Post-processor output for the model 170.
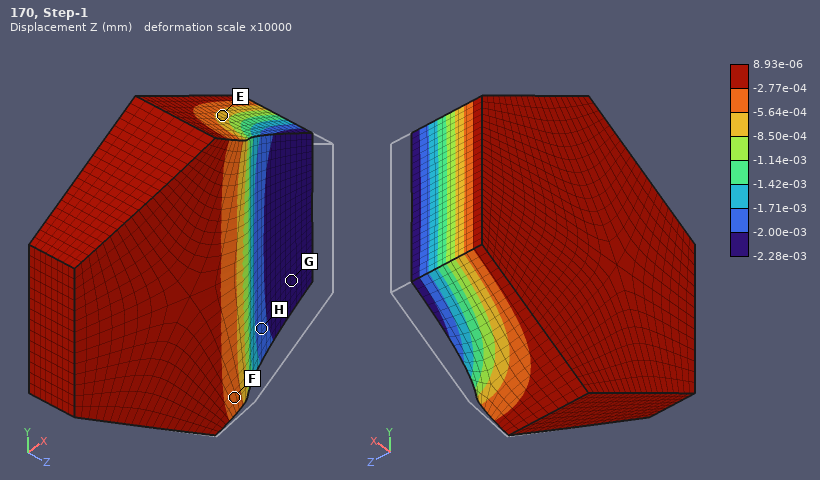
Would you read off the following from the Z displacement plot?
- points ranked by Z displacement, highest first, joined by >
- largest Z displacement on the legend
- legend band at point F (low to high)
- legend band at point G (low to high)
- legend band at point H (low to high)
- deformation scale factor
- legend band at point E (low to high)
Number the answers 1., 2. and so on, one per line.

1. F > E > H > G
2. 8.93e-06 mm
3. -5.64e-04 to -2.77e-04 mm
4. -2.28e-03 to -2.00e-03 mm
5. -2.00e-03 to -1.71e-03 mm
6. 10000
7. -8.50e-04 to -5.64e-04 mm
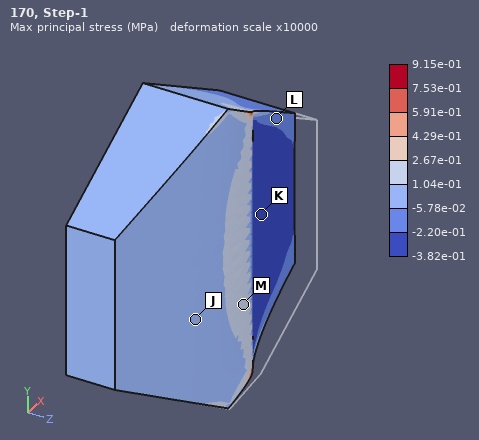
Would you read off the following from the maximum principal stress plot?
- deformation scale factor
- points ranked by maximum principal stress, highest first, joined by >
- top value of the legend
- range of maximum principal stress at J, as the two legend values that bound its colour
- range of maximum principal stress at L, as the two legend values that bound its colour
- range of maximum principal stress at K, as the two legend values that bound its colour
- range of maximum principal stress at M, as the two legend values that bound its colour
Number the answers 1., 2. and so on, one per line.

1. 10000
2. M > J > L > K
3. 9.15e-01 MPa
4. -5.78e-02 to 1.04e-01 MPa
5. -2.20e-01 to -5.78e-02 MPa
6. -3.82e-01 to -2.20e-01 MPa
7. 1.04e-01 to 2.67e-01 MPa
